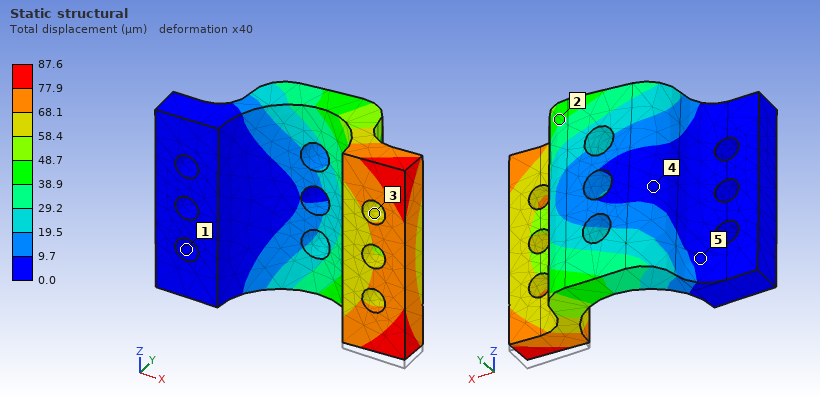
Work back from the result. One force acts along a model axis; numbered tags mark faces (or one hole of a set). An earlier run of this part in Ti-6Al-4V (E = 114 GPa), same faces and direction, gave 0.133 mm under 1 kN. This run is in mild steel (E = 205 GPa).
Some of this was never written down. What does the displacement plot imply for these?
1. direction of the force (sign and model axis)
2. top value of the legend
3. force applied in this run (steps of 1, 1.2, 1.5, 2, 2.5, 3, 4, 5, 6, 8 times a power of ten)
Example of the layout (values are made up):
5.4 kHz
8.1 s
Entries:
+Z
87.6 µm
1.2 kN
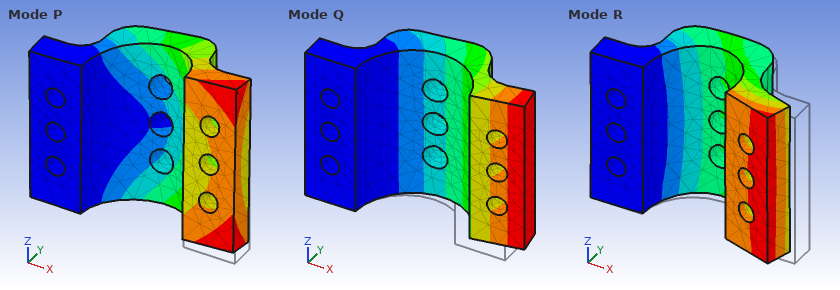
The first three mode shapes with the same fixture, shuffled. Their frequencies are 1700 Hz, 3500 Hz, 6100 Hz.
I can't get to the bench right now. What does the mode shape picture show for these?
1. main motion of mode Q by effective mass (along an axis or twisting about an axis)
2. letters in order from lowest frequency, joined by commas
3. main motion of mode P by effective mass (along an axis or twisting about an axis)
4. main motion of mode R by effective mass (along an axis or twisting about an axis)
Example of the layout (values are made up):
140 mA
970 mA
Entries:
along Y
Q, P, R
along Z
along X
